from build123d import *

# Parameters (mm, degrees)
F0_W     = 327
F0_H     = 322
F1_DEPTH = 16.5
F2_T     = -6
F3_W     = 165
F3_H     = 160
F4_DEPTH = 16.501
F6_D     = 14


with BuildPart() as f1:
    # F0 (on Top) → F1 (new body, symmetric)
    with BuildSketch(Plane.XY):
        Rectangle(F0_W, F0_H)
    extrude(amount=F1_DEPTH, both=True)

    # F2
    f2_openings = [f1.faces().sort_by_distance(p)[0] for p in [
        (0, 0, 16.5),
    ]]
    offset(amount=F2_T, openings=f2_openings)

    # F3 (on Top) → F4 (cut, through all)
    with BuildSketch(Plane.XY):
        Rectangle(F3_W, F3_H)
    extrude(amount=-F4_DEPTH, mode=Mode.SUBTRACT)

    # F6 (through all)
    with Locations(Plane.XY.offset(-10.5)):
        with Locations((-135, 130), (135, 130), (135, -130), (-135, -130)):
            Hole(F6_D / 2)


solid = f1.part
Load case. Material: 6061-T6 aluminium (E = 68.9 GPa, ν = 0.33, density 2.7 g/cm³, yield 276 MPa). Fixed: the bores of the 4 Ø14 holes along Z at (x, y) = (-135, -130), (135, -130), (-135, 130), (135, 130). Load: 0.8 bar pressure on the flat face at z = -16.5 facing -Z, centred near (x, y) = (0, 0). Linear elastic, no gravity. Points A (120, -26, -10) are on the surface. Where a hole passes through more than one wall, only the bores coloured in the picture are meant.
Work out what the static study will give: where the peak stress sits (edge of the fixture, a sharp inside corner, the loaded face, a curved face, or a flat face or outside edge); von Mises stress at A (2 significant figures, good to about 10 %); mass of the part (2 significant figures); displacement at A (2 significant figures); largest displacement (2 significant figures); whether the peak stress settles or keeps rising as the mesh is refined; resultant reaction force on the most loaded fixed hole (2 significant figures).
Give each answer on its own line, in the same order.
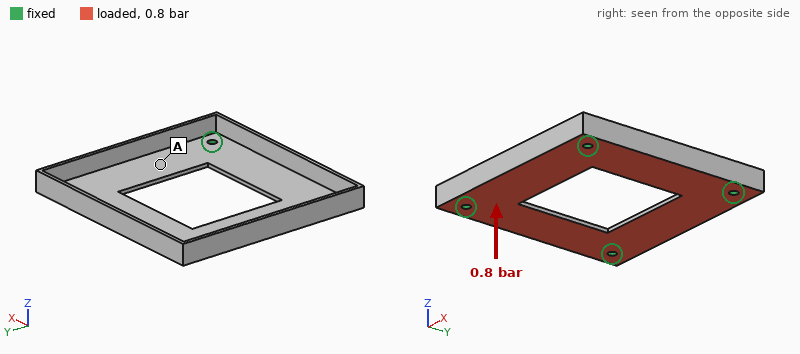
edge of the fixture
12 MPa
1.8 kg
0.37 mm
0.74 mm
keeps rising
1.8 kN
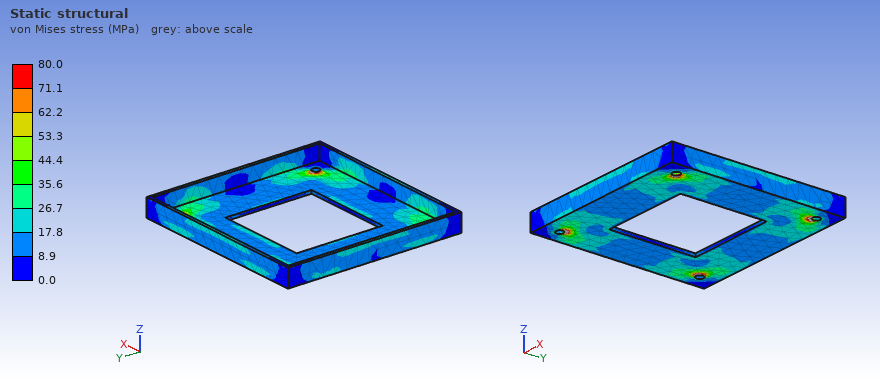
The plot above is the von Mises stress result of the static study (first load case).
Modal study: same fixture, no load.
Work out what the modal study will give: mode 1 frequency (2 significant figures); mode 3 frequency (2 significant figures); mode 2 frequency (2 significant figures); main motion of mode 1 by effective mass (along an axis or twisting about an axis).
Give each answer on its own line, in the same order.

540 Hz
720 Hz
700 Hz
along Z
